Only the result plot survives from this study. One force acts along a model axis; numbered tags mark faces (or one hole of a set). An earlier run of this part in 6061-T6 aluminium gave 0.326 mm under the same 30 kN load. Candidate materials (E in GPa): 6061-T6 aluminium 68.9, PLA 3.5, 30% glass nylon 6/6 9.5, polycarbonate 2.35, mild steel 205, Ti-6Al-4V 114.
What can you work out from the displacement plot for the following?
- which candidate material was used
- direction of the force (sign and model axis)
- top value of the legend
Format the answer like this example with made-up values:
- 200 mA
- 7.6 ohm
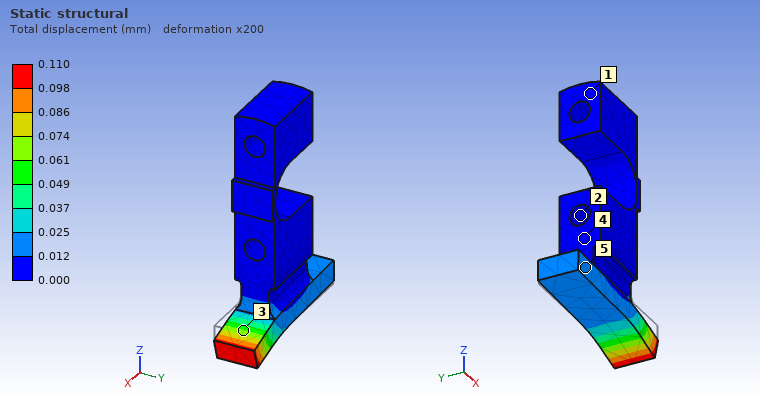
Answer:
- mild steel
- -Z
- 0.110 mm
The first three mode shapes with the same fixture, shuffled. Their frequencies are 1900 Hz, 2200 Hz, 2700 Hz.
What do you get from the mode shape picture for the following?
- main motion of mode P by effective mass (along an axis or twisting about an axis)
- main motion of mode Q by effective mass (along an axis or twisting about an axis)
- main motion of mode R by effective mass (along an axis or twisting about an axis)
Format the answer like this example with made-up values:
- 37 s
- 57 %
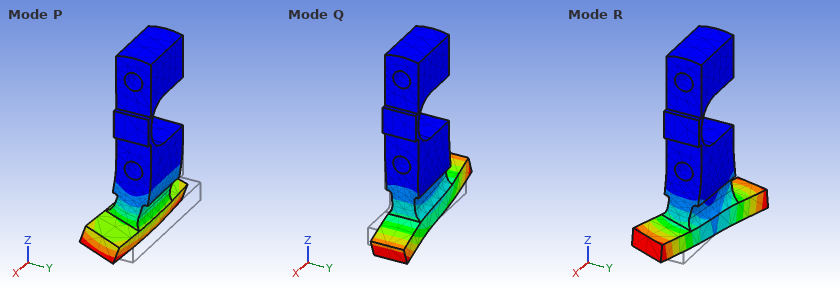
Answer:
- along Y
- along X
- twisting about Z
